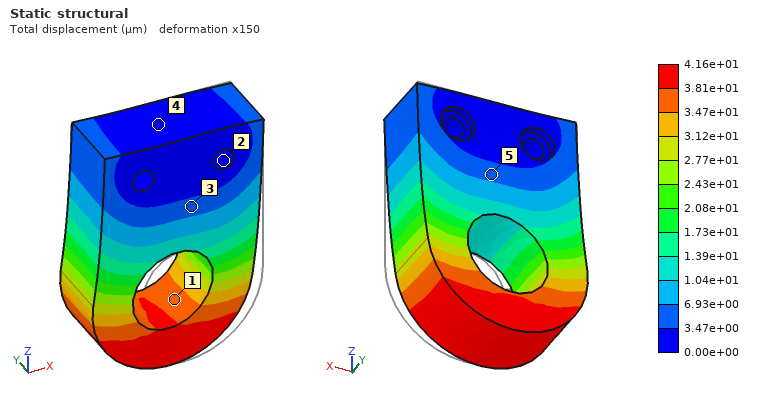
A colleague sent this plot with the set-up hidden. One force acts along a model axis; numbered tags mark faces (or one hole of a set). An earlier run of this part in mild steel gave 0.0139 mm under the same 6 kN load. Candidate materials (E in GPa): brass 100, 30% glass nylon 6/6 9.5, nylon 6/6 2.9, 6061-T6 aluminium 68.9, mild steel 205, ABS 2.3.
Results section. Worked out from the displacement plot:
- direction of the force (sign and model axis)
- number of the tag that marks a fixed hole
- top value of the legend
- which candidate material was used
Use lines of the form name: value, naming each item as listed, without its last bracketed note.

direction of the force: -X
number of the tag that marks a fixed hole: 2
top value of the legend: 4.16e+01 µm
which candidate material was used: 6061-T6 aluminium
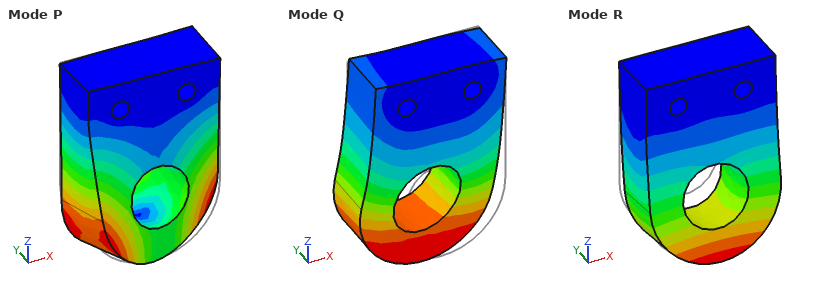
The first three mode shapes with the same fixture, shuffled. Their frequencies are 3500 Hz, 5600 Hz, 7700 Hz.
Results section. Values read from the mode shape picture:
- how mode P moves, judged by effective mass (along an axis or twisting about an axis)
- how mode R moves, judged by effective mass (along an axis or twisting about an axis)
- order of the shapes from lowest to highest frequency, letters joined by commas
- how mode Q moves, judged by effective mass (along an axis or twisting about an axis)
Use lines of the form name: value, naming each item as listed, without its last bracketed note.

how mode P moves, judged by effective mass: twisting about Z
how mode R moves, judged by effective mass: along Y
order of the shapes from lowest to highest frequency, letters joined by commas: R, Q, P
how mode Q moves, judged by effective mass: along X
